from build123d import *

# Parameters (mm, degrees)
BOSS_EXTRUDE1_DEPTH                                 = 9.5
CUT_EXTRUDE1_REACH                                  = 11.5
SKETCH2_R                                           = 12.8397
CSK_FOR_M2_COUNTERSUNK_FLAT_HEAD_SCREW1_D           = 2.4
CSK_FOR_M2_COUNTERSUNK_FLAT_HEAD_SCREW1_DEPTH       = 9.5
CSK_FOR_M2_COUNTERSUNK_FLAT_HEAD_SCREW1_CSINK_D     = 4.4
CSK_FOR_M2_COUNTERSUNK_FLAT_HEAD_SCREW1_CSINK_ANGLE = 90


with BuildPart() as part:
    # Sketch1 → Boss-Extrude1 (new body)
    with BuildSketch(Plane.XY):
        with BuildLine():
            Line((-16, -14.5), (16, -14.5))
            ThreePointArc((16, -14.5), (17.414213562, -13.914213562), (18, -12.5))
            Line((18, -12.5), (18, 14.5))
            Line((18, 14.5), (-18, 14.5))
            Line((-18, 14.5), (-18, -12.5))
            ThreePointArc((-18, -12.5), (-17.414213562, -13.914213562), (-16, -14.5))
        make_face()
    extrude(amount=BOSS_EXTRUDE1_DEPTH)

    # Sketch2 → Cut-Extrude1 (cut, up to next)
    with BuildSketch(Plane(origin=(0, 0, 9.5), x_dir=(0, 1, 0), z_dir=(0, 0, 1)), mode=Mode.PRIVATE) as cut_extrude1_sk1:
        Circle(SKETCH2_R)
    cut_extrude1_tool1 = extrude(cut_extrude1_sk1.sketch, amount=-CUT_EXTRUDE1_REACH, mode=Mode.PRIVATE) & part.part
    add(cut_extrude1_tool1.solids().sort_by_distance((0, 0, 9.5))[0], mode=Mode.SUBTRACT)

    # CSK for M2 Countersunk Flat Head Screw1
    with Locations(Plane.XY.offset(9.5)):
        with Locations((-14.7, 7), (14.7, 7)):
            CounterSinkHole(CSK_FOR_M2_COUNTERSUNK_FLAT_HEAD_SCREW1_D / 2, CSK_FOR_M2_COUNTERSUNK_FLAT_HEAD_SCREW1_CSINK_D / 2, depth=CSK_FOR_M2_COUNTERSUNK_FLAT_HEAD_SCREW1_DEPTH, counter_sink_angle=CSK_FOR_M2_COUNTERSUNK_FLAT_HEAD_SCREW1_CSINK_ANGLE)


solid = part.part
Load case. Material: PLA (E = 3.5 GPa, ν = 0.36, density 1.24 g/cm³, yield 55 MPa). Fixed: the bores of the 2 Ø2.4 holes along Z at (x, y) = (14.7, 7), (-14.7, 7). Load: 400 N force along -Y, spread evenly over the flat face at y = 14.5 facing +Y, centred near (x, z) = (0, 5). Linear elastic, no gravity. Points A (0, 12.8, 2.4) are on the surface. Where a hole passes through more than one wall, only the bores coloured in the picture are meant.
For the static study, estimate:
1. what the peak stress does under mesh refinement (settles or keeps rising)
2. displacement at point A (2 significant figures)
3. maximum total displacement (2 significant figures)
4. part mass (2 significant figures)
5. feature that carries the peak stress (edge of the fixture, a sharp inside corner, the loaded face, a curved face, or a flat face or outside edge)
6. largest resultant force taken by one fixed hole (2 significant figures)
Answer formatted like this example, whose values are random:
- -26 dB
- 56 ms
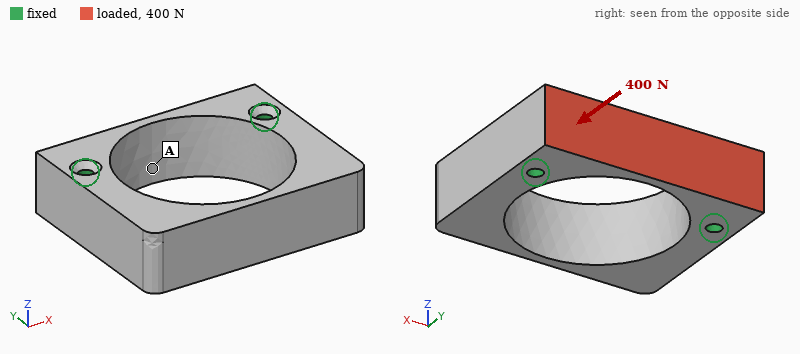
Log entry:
- keeps rising
- 72 µm
- 77 µm
- 6.1 g
- edge of the fixture
- 230 N
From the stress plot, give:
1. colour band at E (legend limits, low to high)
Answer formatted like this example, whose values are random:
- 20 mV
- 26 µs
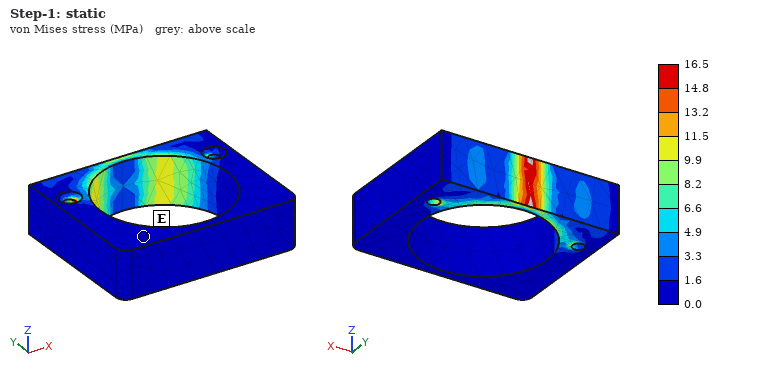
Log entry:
- 0.0 to 1.6 MPa
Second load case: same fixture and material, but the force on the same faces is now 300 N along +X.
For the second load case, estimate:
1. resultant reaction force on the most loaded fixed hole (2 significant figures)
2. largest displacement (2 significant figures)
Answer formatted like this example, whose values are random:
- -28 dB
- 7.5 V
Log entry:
- 150 N
- 46 µm
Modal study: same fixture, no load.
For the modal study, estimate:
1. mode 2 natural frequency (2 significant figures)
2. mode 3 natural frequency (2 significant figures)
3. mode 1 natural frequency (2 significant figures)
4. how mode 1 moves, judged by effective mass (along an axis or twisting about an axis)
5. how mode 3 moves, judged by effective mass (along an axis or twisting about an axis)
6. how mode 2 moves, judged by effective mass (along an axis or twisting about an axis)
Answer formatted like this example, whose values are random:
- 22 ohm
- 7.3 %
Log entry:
- 3200 Hz
- 4700 Hz
- 2900 Hz
- along X
- twisting about Y
- along Z
